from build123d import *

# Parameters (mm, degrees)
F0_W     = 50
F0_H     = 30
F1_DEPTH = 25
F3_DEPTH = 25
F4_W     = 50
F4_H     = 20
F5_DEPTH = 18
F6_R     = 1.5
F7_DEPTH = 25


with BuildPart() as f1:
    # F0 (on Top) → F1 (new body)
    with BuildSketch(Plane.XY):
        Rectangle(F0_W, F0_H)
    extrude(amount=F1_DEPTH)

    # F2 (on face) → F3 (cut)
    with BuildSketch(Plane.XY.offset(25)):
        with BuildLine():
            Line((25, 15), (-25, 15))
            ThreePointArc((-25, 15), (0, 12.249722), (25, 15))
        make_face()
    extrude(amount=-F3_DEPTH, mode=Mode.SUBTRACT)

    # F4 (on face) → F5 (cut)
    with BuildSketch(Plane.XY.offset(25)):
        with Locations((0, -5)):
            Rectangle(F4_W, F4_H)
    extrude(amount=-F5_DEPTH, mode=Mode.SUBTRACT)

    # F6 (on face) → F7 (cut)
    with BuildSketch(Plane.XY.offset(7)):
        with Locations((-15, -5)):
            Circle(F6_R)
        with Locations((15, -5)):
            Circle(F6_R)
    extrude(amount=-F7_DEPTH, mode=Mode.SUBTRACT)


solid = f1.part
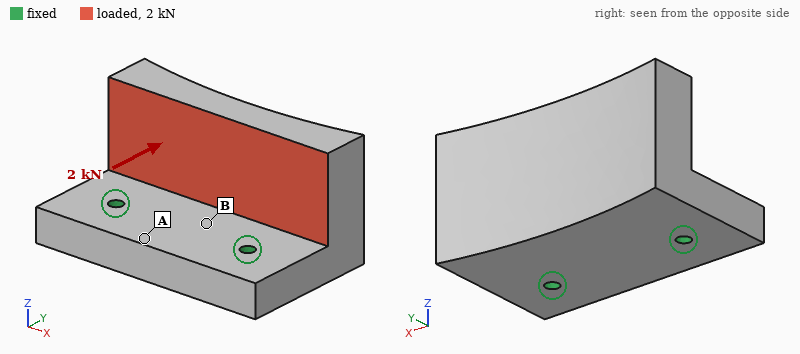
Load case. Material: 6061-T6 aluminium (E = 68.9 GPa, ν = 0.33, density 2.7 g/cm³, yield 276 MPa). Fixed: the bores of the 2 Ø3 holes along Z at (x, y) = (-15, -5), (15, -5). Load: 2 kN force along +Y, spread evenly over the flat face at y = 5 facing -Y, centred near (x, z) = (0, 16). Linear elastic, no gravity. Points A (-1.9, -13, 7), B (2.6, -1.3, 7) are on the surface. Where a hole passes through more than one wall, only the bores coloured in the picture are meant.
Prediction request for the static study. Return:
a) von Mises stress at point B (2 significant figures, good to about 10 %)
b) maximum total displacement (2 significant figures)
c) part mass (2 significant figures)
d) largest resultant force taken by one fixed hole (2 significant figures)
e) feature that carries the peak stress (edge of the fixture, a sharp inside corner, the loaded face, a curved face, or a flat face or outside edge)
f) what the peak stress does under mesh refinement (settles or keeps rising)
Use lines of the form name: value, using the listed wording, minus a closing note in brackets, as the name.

von Mises stress at point B: 39 MPa
maximum total displacement: 0.12 mm
part mass: 46 g
largest resultant force taken by one fixed hole: 1.0 kN
feature that carries the peak stress: edge of the fixture
what the peak stress does under mesh refinement: keeps rising
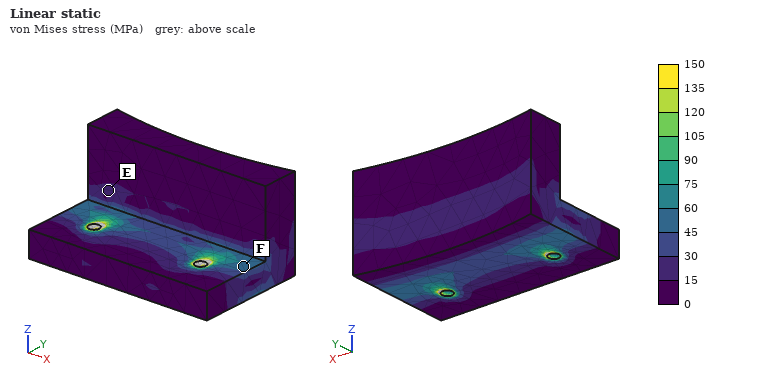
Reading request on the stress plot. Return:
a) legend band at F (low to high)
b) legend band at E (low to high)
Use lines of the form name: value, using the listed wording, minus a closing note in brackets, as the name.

legend band at F: 45 to 60 MPa
legend band at E: 15 to 30 MPa
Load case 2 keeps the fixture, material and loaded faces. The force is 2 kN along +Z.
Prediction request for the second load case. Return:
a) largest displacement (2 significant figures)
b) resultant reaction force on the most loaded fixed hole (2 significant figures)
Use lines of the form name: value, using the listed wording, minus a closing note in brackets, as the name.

largest displacement: 44 µm
resultant reaction force on the most loaded fixed hole: 1.0 kN
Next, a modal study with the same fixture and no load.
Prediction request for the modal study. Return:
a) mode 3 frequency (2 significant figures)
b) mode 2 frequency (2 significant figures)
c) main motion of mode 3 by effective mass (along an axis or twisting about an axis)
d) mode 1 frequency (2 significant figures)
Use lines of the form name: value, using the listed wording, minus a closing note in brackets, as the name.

mode 3 frequency: 13 kHz
mode 2 frequency: 8200 Hz
main motion of mode 3 by effective mass: along X
mode 1 frequency: 4800 Hz
